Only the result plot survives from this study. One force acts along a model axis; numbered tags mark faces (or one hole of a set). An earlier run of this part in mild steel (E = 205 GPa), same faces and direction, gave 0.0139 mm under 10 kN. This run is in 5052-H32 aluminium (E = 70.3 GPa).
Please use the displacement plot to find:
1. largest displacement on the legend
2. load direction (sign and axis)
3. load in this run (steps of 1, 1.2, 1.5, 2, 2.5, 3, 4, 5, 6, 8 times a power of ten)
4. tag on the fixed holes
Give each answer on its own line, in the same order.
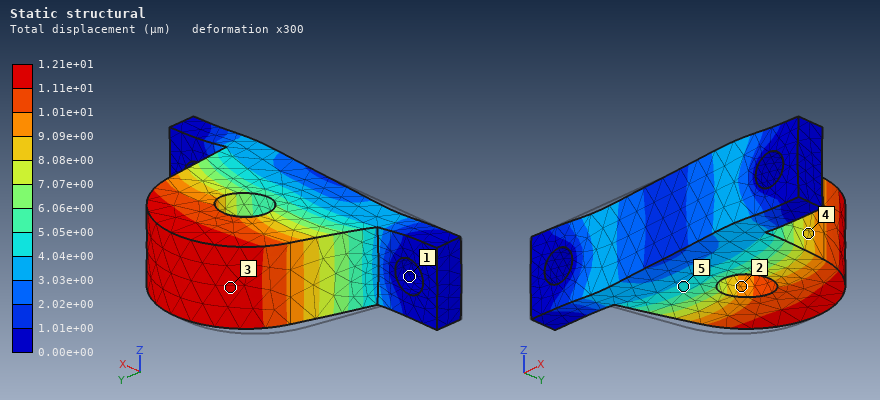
1.21e+01 µm
+X
3 kN
1
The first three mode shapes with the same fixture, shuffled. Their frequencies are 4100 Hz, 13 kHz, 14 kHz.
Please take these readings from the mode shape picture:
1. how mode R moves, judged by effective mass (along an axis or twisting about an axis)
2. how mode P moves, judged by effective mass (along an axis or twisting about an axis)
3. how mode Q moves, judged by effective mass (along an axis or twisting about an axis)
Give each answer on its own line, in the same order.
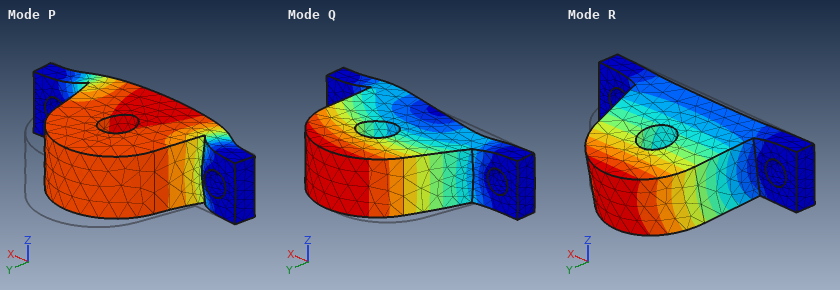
along Z
along Y
along X
